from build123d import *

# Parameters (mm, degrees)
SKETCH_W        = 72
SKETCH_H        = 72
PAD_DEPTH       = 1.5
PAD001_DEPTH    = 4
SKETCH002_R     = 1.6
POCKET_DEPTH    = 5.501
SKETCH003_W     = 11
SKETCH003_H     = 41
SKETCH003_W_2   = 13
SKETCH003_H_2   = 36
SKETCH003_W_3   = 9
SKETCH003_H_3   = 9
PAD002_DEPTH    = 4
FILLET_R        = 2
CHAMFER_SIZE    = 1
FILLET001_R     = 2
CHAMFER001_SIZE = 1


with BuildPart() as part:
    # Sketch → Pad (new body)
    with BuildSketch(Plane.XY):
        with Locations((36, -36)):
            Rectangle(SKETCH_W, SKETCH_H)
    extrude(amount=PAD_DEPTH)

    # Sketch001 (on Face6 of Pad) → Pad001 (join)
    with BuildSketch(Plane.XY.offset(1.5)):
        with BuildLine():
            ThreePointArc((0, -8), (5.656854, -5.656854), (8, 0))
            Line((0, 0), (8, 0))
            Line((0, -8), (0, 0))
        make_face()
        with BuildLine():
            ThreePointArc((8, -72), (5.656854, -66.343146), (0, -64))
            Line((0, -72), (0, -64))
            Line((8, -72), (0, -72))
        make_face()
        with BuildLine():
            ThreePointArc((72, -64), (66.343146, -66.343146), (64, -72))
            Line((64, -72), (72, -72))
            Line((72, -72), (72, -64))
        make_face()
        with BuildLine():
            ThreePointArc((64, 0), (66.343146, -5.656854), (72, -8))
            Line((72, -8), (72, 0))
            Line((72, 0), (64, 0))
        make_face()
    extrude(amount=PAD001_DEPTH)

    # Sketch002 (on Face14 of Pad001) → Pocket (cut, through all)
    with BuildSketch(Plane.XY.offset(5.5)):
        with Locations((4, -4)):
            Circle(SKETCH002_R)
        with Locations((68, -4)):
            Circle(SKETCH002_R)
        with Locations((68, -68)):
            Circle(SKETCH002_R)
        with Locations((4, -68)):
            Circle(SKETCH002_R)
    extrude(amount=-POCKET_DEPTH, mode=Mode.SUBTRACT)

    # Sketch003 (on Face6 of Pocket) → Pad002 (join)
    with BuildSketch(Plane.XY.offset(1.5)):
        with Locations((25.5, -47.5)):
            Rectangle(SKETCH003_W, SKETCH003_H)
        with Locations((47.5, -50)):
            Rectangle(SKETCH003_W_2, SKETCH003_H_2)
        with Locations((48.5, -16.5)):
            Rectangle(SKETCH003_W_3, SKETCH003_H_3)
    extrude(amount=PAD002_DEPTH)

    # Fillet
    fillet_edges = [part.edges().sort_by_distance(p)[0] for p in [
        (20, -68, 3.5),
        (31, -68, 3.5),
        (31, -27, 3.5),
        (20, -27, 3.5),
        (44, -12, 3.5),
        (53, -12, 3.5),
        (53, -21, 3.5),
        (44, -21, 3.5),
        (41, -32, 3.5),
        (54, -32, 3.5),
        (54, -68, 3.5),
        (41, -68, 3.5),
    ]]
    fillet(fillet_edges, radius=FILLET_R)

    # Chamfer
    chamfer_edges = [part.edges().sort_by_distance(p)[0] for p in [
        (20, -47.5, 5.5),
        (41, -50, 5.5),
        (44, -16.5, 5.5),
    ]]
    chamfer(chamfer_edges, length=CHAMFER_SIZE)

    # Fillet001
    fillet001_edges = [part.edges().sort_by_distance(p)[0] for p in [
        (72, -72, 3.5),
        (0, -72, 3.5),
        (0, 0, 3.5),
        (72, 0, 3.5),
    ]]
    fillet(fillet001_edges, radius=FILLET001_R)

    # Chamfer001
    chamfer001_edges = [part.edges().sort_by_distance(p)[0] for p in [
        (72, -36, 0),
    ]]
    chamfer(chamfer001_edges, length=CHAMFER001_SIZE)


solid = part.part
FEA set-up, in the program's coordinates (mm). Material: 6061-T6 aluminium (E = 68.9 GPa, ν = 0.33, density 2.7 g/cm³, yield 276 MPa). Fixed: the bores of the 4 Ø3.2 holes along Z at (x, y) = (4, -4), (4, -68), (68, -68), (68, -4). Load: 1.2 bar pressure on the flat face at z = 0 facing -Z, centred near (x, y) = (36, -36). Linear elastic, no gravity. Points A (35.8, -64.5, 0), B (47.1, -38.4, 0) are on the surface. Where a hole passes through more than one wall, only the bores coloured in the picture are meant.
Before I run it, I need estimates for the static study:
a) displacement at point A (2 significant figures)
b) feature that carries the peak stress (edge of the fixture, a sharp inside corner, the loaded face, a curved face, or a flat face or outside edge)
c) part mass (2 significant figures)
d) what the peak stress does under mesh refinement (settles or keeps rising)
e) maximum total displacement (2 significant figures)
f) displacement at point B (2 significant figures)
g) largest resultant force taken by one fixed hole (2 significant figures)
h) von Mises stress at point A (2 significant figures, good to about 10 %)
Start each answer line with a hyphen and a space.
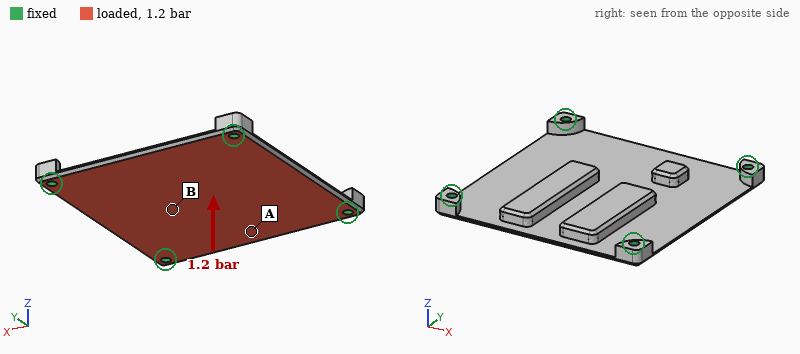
- 0.27 mm
- edge of the fixture
- 33 g
- keeps rising
- 0.50 mm
- 0.39 mm
- 150 N
- 65 MPa
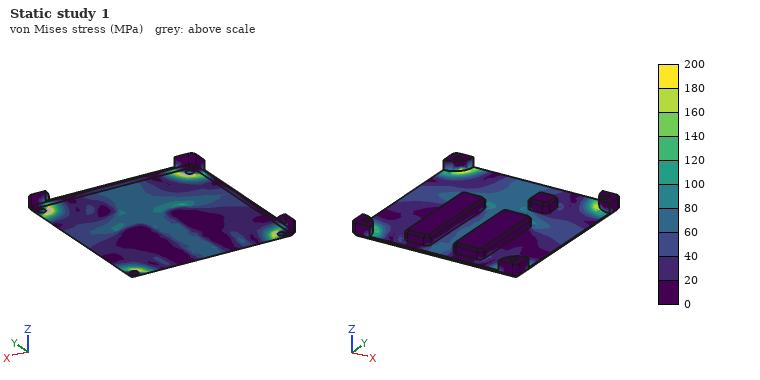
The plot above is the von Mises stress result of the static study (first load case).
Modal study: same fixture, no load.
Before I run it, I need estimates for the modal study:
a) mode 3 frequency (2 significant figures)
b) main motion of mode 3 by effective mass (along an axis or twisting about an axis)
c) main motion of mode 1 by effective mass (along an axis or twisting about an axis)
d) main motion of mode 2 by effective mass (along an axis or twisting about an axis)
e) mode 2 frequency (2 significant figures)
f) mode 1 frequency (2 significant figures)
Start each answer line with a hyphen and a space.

- 2600 Hz
- twisting about Y
- along Z
- twisting about X
- 2300 Hz
- 1200 Hz
